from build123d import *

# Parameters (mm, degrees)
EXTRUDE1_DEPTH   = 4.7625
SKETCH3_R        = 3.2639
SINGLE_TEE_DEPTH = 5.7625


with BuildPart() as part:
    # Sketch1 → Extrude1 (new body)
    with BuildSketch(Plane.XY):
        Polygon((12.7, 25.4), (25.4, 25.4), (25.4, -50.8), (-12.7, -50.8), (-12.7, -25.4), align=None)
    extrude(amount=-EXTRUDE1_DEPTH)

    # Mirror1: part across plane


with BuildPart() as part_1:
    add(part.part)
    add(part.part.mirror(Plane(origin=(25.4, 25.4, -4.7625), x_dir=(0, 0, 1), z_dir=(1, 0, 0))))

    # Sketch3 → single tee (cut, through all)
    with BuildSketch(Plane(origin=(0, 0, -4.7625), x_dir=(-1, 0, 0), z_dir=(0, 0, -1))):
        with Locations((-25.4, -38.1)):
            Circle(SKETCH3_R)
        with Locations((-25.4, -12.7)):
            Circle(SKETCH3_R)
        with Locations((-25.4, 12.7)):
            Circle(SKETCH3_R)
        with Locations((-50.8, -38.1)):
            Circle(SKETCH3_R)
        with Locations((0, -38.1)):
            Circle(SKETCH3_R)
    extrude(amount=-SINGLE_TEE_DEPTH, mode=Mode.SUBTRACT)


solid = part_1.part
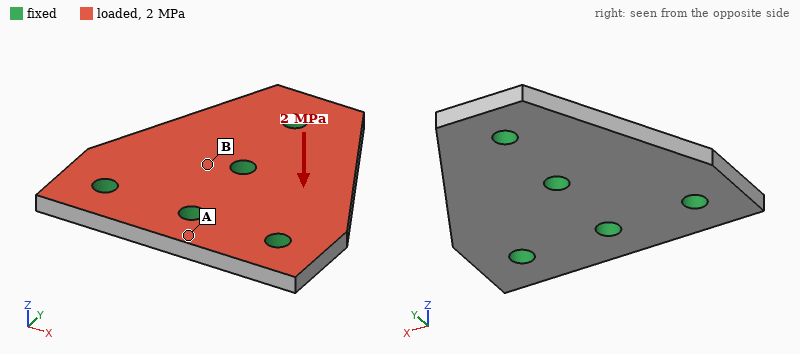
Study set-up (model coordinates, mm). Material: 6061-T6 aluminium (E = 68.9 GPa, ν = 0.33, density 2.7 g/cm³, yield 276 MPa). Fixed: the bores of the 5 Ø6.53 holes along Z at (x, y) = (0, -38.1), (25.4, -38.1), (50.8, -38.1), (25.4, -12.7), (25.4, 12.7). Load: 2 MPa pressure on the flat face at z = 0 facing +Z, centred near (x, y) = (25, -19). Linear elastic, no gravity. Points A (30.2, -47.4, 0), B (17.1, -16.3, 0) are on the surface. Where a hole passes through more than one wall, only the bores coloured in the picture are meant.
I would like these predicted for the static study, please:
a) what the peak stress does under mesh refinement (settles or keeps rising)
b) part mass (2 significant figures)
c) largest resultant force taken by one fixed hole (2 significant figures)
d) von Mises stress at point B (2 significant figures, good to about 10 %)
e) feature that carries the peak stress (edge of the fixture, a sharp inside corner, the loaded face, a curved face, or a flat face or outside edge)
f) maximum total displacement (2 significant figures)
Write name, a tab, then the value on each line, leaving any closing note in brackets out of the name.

what the peak stress does under mesh refinement	keeps rising
part mass	56 g
largest resultant force taken by one fixed hole	2.2 kN
von Mises stress at point B	40 MPa
feature that carries the peak stress	edge of the fixture
maximum total displacement	92 µm
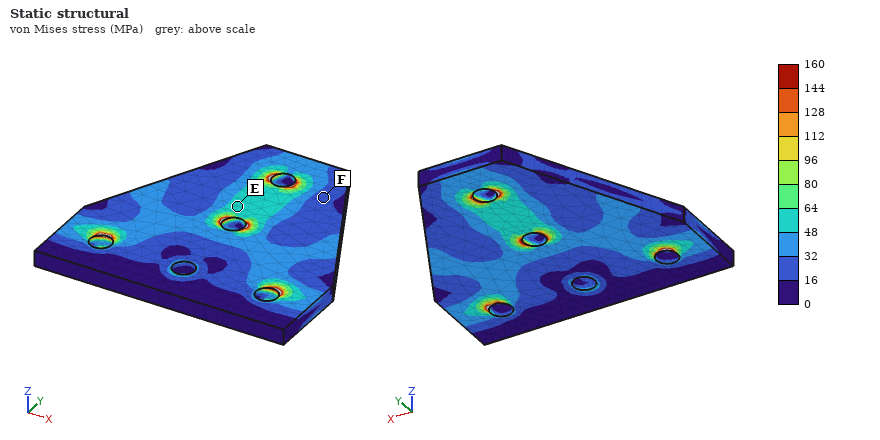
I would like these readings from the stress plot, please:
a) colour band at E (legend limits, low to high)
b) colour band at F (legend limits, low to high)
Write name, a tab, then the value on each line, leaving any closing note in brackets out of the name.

colour band at E	48 to 64 MPa
colour band at F	16 to 32 MPa
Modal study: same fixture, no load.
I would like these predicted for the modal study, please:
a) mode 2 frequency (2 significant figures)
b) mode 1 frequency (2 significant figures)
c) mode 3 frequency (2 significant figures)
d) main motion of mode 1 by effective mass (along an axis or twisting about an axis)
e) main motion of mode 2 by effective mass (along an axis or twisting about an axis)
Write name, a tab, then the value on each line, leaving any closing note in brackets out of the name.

mode 2 frequency	8800 Hz
mode 1 frequency	8400 Hz
mode 3 frequency	15 kHz
main motion of mode 1 by effective mass	twisting about Y
main motion of mode 2 by effective mass	along Z
